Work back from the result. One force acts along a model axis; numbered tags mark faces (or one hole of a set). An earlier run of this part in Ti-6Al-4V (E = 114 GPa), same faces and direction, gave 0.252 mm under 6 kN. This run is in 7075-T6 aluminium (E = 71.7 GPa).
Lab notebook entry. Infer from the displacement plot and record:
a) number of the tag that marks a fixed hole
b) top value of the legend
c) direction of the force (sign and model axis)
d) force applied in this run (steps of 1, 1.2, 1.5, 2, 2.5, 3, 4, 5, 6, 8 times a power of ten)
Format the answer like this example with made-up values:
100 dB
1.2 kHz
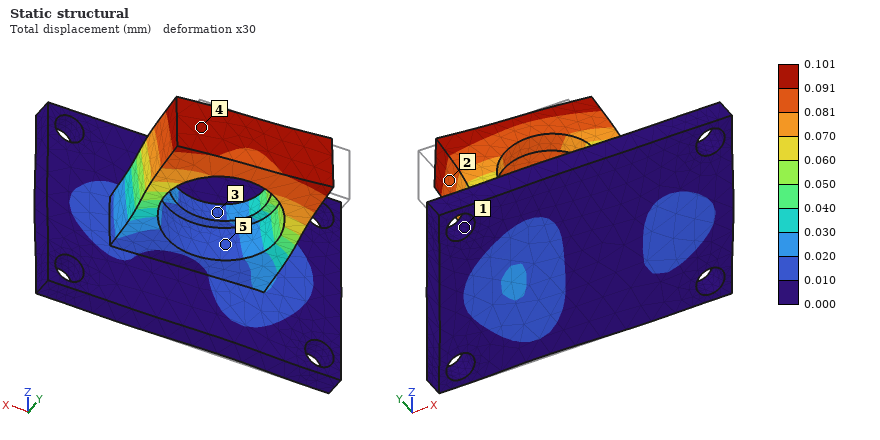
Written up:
1
0.101 mm
+X
1.5 kN
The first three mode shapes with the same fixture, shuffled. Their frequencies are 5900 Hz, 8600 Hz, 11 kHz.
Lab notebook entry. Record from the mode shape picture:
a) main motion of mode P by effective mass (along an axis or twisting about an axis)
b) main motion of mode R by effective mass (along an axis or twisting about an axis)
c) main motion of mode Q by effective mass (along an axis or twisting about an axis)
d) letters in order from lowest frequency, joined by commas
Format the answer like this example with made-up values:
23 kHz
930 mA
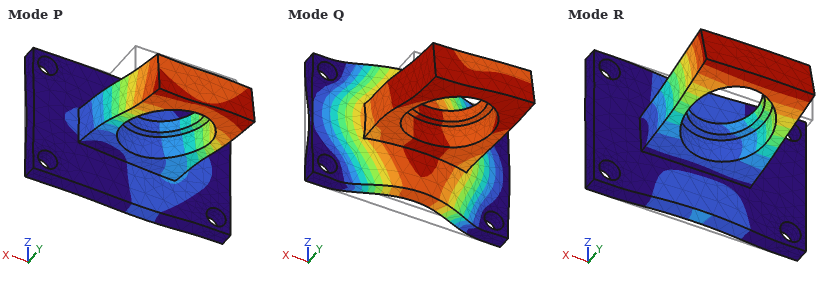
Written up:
along X
along Z
along Y
R, P, Q
